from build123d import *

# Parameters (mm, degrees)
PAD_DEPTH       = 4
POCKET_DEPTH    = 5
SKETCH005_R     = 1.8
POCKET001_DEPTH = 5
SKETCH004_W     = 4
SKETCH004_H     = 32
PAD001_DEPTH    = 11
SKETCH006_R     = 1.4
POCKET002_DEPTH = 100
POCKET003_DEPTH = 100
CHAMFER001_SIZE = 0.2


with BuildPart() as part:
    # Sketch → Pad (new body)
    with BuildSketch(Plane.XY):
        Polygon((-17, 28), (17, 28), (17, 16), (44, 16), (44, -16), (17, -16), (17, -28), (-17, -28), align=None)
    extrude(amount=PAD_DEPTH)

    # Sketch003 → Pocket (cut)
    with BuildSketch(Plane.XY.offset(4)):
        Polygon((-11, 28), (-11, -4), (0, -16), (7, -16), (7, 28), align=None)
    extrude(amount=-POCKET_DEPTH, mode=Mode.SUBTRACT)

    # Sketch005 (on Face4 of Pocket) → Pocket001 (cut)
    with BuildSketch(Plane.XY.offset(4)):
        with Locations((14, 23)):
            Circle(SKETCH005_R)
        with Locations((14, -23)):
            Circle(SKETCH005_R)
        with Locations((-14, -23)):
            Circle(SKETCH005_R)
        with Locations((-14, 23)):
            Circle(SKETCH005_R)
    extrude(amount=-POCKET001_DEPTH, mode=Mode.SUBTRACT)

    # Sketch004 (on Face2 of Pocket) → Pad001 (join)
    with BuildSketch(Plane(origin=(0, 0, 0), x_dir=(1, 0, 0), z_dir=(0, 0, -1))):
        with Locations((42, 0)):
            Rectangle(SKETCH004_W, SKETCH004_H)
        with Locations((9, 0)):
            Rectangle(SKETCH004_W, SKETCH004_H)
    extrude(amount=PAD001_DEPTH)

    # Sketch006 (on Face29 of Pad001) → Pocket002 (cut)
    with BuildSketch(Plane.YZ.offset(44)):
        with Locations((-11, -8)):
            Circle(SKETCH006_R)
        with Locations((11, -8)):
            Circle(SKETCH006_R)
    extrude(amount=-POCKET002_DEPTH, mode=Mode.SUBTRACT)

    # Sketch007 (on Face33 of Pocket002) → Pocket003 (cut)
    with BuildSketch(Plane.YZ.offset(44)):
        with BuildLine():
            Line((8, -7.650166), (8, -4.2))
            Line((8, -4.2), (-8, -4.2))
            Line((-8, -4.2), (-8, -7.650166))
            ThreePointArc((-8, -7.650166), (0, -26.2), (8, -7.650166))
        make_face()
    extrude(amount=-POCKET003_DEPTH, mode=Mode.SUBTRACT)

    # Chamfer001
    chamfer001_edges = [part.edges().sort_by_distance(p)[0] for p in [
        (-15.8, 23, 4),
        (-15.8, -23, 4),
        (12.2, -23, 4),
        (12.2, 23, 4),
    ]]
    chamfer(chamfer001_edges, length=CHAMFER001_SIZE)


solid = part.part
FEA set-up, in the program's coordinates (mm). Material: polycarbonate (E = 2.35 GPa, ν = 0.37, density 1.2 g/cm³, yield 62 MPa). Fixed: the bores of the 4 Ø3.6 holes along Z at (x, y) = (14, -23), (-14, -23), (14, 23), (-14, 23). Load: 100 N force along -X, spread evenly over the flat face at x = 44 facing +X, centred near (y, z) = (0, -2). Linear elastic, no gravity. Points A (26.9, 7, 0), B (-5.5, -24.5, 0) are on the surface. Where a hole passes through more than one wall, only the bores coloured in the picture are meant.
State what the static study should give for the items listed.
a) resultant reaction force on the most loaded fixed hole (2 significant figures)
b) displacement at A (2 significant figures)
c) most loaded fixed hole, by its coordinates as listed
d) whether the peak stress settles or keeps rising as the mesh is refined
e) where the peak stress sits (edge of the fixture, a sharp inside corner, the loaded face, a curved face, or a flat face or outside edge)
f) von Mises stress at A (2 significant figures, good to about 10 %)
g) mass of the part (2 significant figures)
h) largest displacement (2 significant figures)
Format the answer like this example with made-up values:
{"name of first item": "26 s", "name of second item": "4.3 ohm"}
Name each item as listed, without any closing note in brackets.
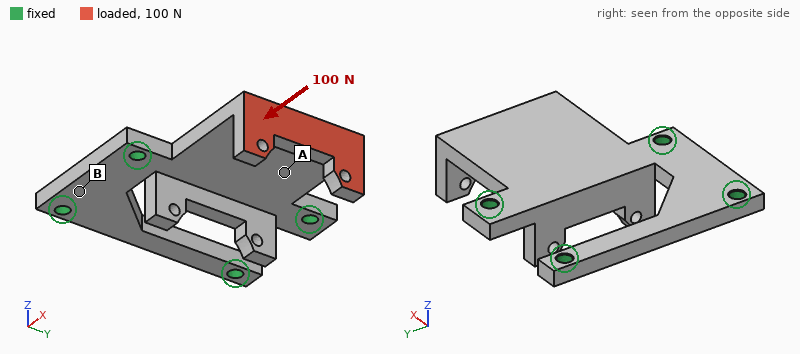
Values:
{"resultant reaction force on the most loaded fixed hole": "47 N", "displacement at A": "0.26 mm", "most loaded fixed hole, by its coordinates as listed": "(14, 23)", "whether the peak stress settles or keeps rising as the mesh is refined": "keeps rising", "where the peak stress sits": "edge of the fixture", "von Mises stress at A": "4.9 MPa", "mass of the part": "12 g", "largest displacement": "0.96 mm"}
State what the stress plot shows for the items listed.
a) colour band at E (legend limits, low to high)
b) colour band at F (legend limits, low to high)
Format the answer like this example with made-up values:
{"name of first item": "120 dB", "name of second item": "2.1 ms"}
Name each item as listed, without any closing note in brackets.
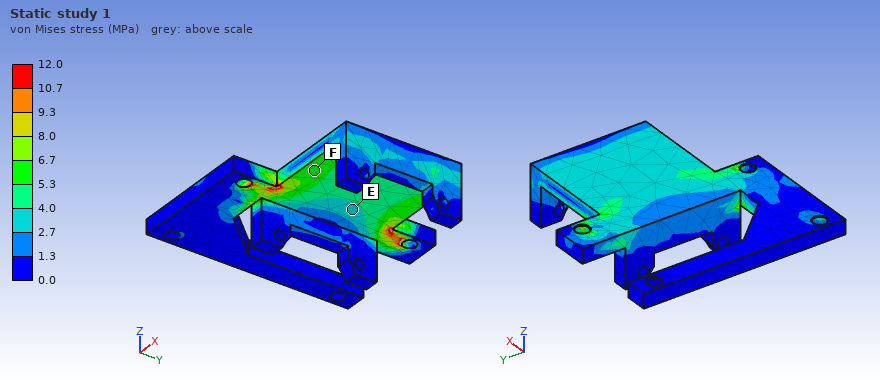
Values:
{"colour band at E": "2.7 to 4.0 MPa", "colour band at F": "5.3 to 6.7 MPa"}
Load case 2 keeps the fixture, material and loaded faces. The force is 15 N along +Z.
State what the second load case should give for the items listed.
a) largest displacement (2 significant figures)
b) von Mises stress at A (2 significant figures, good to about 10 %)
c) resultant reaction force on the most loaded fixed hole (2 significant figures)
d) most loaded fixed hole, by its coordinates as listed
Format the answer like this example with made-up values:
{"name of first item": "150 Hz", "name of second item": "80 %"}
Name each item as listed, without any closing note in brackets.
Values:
{"largest displacement": "0.85 mm", "von Mises stress at A": "3.1 MPa", "resultant reaction force on the most loaded fixed hole": "13 N", "most loaded fixed hole, by its coordinates as listed": "(14, -23)"}
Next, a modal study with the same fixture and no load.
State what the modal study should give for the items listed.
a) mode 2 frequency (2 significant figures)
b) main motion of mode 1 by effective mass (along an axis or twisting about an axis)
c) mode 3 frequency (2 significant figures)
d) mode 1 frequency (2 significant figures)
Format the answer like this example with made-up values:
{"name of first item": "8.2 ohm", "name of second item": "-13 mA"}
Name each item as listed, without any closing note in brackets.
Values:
{"mode 2 frequency": "1400 Hz", "main motion of mode 1 by effective mass": "along Z", "mode 3 frequency": "2500 Hz", "mode 1 frequency": "460 Hz"}
